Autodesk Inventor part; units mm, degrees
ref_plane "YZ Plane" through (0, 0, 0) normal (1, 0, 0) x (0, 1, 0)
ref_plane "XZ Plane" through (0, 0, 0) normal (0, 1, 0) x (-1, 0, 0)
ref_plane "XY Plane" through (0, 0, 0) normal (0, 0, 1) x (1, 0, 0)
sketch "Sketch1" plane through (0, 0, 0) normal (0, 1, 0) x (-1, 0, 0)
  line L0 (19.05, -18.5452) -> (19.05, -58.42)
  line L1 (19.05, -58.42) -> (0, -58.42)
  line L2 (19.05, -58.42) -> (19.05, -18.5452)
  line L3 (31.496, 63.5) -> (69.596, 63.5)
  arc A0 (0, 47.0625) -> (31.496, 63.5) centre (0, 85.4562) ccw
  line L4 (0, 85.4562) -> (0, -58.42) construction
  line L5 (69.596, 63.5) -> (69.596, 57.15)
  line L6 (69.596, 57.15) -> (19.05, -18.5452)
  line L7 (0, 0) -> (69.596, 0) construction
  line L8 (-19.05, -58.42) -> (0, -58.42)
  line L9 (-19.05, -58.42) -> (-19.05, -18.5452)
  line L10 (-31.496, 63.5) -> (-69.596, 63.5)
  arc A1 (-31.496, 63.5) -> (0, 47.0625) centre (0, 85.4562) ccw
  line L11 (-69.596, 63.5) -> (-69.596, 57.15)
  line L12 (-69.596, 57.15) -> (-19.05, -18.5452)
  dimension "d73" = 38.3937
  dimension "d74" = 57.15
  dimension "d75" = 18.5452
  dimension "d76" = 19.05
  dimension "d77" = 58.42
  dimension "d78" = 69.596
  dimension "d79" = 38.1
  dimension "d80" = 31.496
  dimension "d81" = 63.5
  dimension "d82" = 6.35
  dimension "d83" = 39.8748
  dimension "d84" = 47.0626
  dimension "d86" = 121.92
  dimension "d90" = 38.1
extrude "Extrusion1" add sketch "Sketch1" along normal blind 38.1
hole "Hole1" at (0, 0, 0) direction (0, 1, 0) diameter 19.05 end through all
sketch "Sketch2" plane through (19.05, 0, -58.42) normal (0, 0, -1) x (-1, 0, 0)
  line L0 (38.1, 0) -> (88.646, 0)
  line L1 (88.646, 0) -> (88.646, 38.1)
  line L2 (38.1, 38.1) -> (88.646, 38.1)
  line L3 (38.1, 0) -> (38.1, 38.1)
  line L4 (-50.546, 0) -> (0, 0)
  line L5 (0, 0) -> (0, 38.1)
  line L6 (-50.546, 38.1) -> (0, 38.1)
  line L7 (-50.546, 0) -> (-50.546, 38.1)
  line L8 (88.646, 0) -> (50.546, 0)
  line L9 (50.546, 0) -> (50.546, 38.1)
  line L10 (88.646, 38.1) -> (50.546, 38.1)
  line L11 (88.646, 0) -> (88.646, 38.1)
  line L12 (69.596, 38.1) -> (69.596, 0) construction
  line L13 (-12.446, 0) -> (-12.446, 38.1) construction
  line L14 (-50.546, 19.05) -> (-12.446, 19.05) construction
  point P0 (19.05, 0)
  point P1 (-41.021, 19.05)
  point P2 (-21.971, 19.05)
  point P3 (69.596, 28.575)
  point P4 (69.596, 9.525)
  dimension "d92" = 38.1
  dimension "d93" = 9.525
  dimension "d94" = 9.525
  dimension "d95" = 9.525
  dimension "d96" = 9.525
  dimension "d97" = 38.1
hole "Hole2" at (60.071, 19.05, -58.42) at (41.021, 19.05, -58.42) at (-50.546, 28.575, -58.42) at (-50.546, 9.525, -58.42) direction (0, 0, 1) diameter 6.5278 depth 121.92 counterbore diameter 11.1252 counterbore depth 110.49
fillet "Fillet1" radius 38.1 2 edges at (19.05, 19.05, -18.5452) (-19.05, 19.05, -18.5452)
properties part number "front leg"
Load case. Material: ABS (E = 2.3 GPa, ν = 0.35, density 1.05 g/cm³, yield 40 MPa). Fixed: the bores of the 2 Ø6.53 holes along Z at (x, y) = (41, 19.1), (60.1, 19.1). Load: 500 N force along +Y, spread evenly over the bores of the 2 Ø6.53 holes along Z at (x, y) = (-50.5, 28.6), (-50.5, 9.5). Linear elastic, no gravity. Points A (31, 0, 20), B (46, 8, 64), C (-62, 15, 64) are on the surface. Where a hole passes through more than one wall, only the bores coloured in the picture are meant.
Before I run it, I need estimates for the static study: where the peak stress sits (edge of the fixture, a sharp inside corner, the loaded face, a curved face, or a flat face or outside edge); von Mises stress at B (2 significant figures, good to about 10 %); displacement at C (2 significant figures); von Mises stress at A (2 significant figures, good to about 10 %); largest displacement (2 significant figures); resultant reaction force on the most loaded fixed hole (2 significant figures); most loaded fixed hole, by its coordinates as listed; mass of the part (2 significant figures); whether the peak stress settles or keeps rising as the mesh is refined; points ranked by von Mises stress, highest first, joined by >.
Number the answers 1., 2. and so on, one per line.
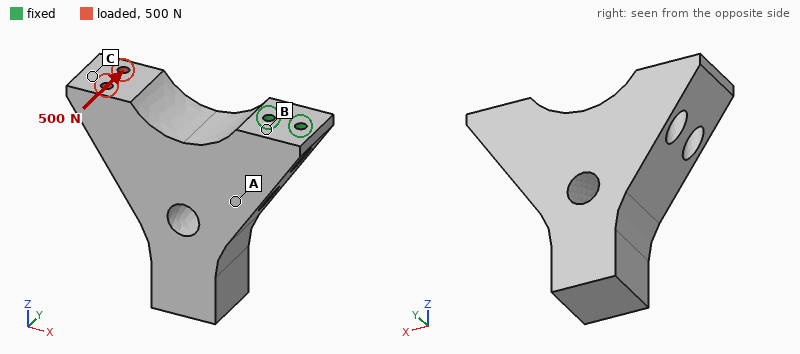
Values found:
1. edge of the fixture
2. 6.4 MPa
3. 1.3 mm
4. 3.1 MPa
5. 1.4 mm
6. 2.3 kN
7. (41, 19.1)
8. 310 g
9. keeps rising
10. B > A > C
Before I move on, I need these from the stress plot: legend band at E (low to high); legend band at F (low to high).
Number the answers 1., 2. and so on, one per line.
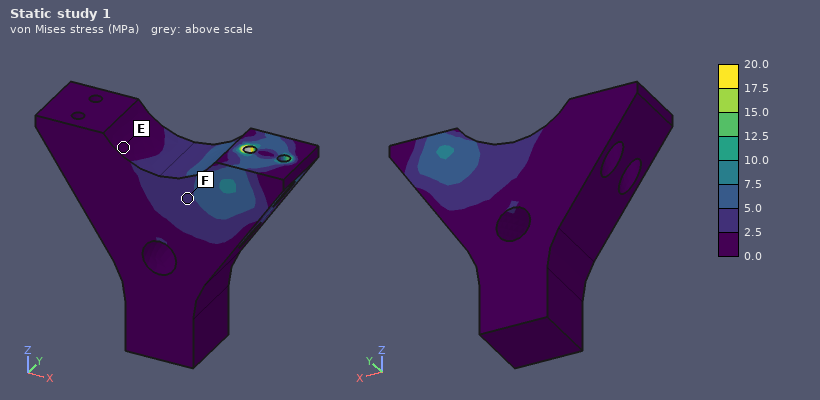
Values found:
1. 0.0 to 2.5 MPa
2. 2.5 to 5.0 MPa
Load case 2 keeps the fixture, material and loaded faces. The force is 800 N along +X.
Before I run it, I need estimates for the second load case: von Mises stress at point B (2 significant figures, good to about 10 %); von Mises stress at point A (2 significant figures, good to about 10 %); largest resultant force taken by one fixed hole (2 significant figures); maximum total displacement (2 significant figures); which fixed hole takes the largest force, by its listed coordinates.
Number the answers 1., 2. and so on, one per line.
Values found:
1. 1.0 MPa
2. 0.51 MPa
3. 590 N
4. 0.28 mm
5. (41, 19.1)
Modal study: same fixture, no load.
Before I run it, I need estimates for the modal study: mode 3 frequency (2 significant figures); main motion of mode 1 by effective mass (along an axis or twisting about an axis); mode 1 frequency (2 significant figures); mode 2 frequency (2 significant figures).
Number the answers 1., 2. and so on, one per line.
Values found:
1. 470 Hz
2. along Y
3. 240 Hz
4. 260 Hz
